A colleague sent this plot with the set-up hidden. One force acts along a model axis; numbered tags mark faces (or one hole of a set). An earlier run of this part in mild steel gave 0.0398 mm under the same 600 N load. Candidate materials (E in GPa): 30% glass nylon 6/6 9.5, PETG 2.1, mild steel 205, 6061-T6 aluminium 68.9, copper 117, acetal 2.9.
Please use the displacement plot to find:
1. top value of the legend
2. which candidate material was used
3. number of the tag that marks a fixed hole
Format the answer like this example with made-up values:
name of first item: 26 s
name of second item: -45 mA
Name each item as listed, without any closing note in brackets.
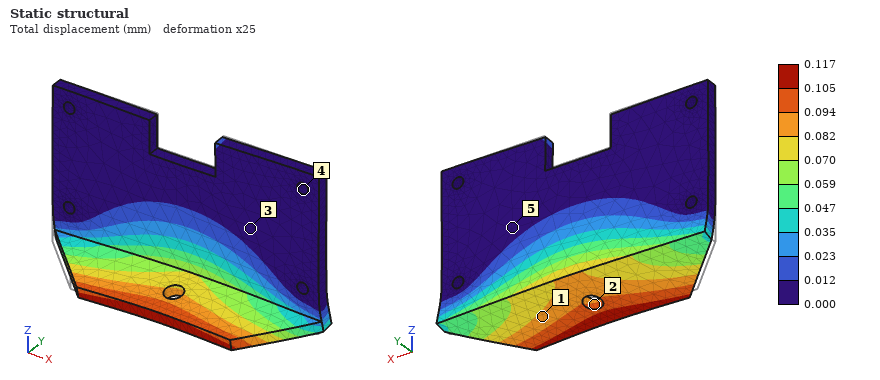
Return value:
top value of the legend: 0.117 mm
which candidate material was used: 6061-T6 aluminium
number of the tag that marks a fixed hole: 4
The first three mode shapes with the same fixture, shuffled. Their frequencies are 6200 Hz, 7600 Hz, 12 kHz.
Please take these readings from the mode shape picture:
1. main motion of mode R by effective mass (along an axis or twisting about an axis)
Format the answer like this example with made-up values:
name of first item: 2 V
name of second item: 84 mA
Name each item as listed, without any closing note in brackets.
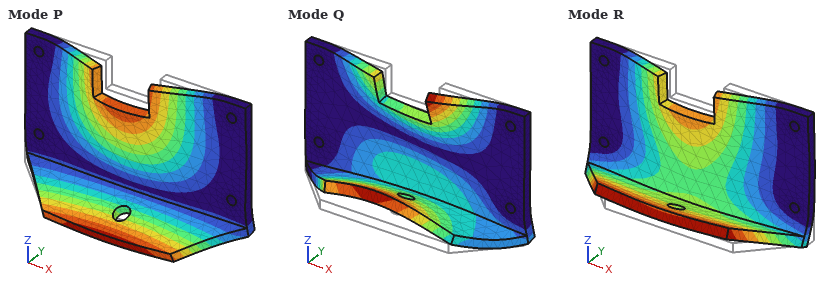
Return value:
main motion of mode R by effective mass: along Y
